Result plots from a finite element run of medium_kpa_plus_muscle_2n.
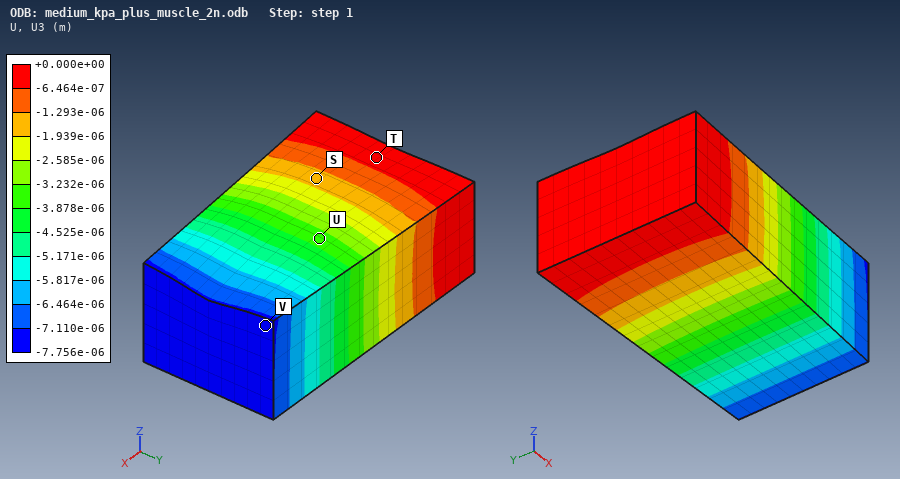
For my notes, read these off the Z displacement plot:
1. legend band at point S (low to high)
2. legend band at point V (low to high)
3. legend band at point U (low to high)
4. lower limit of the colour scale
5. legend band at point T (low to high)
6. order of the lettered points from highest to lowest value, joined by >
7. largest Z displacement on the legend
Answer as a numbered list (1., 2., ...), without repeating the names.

1. -1.939e-06 to -1.293e-06 m
2. -7.756e-06 to -7.110e-06 m
3. -3.878e-06 to -3.232e-06 m
4. -7.756e-06 m
5. -6.464e-07 to +0.000e+00 m
6. T > S > U > V
7. +0.000e+00 m
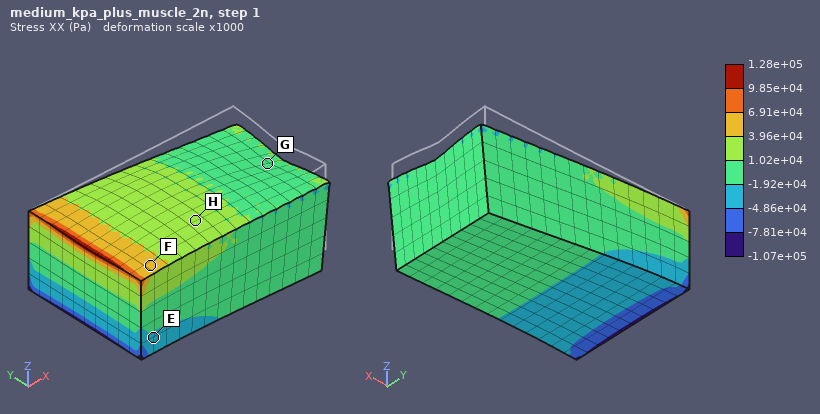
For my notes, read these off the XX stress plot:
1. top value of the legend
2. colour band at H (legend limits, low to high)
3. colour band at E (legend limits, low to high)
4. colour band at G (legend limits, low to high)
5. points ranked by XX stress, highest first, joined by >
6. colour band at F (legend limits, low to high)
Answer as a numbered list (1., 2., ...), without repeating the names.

1. 1.28e+05 Pa
2. 1.02e+04 to 3.96e+04 Pa
3. -4.86e+04 to -1.92e+04 Pa
4. -1.92e+04 to 1.02e+04 Pa
5. F > H > G > E
6. 3.96e+04 to 6.91e+04 Pa
